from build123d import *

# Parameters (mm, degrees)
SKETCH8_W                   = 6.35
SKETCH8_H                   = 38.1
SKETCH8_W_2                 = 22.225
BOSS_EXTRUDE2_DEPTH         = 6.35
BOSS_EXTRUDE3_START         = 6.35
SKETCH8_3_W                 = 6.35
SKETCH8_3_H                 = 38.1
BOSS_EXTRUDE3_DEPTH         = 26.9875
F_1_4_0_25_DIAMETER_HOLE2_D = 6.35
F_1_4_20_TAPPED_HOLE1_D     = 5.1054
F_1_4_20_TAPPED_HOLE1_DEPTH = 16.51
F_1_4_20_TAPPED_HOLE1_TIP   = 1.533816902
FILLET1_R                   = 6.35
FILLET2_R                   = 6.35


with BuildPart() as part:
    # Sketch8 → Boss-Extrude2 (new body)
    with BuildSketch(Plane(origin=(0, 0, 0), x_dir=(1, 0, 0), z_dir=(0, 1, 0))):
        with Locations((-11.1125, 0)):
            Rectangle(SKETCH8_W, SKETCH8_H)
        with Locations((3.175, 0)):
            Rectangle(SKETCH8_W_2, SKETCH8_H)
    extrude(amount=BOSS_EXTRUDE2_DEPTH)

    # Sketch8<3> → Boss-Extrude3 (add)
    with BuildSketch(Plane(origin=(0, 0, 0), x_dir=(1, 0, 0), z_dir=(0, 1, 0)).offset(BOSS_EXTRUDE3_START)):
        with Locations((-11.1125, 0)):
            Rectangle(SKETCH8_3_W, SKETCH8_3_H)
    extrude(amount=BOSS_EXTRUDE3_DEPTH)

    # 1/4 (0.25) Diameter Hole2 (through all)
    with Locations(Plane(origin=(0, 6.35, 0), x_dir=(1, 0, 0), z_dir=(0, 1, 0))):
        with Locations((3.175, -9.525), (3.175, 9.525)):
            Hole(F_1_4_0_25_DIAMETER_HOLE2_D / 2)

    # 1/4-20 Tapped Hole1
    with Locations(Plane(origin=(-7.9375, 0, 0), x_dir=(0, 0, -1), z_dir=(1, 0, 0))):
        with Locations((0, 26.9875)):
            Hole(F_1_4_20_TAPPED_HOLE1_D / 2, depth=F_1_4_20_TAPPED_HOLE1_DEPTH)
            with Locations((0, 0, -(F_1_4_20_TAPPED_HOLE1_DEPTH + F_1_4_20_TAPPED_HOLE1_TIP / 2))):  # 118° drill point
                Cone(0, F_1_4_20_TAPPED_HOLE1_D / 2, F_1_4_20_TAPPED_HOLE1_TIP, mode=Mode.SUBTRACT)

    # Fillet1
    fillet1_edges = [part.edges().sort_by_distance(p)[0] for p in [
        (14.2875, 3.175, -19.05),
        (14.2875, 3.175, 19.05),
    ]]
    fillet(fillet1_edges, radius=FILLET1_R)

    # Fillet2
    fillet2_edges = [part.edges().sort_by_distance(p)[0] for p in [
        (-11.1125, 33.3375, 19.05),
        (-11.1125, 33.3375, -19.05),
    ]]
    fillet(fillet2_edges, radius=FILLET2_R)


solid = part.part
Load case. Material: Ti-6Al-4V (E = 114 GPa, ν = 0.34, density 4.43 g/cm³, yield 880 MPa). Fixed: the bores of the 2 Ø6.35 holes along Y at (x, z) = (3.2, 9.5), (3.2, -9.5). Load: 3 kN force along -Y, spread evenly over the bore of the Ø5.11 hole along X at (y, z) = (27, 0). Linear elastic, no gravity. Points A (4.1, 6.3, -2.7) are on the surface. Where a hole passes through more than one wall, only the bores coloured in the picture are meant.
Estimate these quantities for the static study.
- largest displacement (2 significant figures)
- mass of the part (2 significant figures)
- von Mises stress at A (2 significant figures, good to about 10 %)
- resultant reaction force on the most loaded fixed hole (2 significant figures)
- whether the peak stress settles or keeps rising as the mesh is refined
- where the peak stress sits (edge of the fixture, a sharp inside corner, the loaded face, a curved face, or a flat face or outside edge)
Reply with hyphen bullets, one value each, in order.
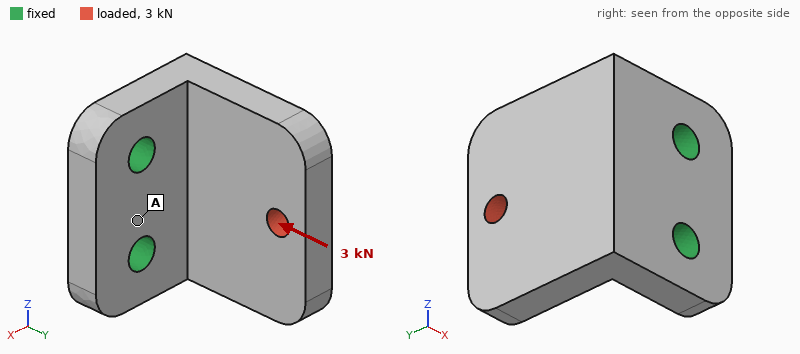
- 93 µm
- 56 g
- 38 MPa
- 1.5 kN
- keeps rising
- edge of the fixture
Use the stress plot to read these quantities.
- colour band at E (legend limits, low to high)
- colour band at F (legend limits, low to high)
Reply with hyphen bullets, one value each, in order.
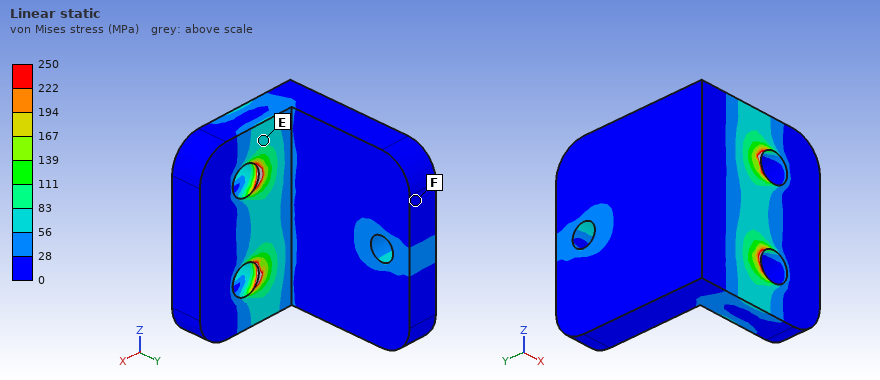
- 56 to 83 MPa
- 0 to 28 MPa
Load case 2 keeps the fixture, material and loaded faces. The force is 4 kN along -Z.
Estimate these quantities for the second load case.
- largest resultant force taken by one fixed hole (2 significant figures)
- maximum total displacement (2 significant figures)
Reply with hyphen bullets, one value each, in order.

- 4.7 kN
- 0.13 mm
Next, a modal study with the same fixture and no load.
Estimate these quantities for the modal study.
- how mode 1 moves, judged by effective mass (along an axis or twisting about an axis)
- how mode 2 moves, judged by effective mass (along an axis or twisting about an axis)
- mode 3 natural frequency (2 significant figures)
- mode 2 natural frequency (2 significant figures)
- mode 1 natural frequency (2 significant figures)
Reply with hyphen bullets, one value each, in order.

- along X
- along Z
- 11 kHz
- 6800 Hz
- 3700 Hz
